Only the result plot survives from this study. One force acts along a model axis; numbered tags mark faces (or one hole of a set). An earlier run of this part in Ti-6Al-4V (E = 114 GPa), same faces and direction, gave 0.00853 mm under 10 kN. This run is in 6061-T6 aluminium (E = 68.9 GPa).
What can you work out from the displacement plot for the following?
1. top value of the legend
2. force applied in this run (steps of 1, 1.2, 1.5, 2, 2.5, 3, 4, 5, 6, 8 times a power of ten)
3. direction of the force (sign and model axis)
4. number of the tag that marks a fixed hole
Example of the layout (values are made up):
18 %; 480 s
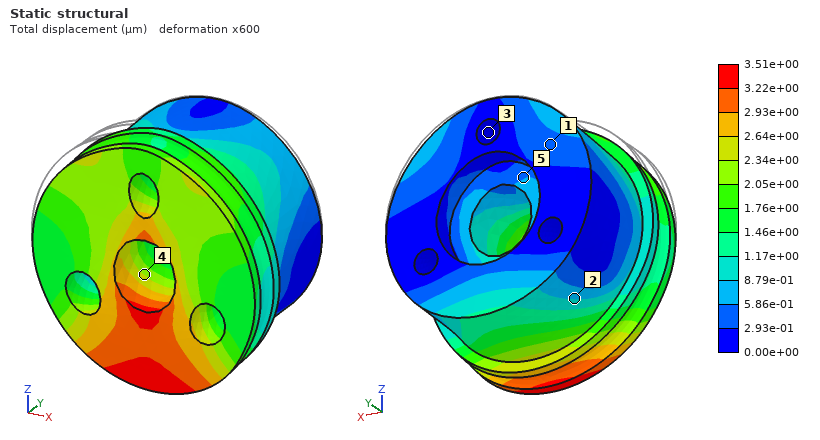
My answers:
3.51e+00 µm; 2.5 kN; -Z; 3
